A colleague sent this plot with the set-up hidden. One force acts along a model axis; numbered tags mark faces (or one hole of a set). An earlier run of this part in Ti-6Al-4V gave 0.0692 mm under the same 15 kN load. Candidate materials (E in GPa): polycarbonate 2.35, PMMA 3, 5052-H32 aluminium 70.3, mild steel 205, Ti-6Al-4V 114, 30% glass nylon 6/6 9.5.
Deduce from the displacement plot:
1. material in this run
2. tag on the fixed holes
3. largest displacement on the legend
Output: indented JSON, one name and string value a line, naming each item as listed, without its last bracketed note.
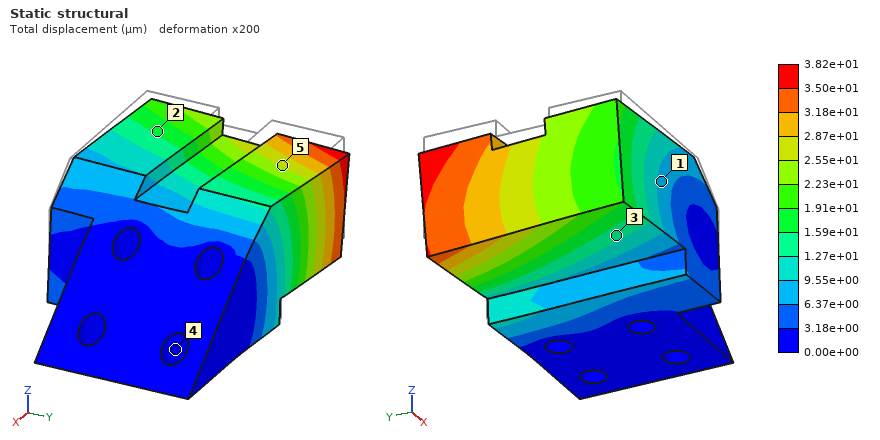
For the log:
{
  "material in this run": "mild steel",
  "tag on the fixed holes": "4",
  "largest displacement on the legend": "3.82e+01 µm"
}
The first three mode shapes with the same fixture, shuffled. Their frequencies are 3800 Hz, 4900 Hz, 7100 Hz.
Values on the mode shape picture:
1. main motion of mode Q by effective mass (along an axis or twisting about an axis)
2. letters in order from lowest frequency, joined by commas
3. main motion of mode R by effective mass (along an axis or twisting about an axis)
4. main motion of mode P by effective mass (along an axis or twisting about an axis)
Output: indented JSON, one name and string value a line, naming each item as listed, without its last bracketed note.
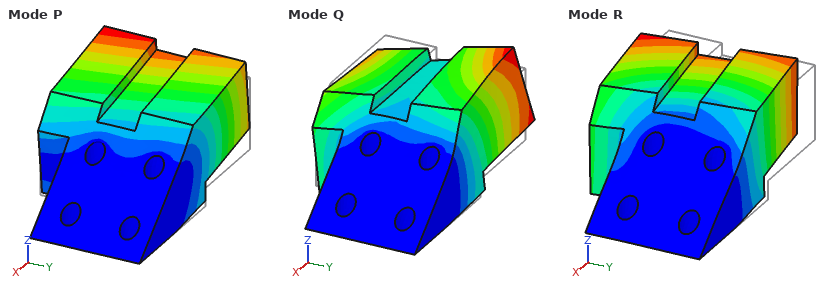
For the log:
{
  "main motion of mode Q by effective mass": "twisting about X",
  "letters in order from lowest frequency, joined by commas": "P, R, Q",
  "main motion of mode R by effective mass": "along Y",
  "main motion of mode P by effective mass": "along Z"
}
